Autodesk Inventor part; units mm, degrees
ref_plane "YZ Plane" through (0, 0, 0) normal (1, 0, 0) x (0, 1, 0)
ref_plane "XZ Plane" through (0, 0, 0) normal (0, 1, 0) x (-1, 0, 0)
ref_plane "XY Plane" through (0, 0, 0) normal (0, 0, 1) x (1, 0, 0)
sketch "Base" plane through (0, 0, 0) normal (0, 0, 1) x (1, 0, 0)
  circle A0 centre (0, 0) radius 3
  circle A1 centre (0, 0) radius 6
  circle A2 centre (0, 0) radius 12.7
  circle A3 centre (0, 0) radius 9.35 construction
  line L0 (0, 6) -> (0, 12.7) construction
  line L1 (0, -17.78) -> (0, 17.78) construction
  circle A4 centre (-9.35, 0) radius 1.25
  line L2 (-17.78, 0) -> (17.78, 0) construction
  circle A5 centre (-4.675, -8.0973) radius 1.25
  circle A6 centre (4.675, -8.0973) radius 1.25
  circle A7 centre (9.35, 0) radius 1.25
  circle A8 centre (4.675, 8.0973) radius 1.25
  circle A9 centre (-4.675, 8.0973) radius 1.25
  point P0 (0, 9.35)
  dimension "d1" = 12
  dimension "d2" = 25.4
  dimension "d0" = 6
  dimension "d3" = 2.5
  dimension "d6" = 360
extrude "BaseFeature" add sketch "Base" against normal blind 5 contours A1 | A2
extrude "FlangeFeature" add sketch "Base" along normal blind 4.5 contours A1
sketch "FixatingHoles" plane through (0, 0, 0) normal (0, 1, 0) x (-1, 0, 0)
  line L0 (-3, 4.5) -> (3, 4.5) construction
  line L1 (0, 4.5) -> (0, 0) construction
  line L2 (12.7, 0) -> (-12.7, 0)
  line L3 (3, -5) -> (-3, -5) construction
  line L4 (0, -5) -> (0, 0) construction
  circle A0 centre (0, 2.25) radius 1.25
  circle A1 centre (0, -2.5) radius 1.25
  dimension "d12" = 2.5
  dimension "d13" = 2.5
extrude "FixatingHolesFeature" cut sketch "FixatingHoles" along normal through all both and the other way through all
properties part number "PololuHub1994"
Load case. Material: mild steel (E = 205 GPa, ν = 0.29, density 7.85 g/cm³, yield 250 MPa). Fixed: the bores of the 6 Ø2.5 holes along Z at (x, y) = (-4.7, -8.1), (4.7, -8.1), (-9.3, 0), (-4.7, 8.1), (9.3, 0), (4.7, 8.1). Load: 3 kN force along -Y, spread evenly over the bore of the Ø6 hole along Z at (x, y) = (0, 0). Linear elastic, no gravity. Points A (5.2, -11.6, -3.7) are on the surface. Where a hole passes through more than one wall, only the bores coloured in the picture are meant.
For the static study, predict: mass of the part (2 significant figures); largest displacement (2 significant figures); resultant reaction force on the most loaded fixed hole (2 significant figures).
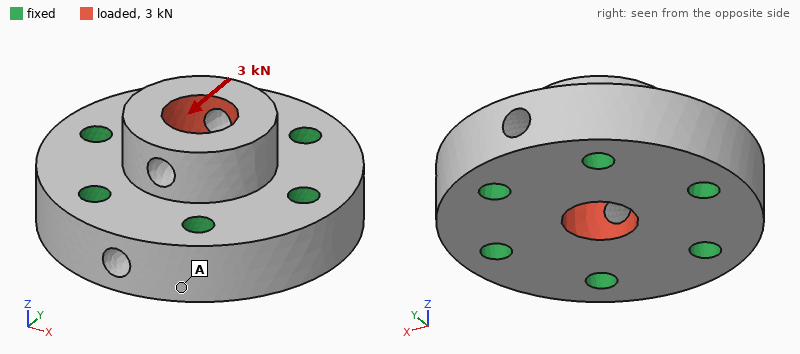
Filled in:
20 g
2.5 µm
690 N
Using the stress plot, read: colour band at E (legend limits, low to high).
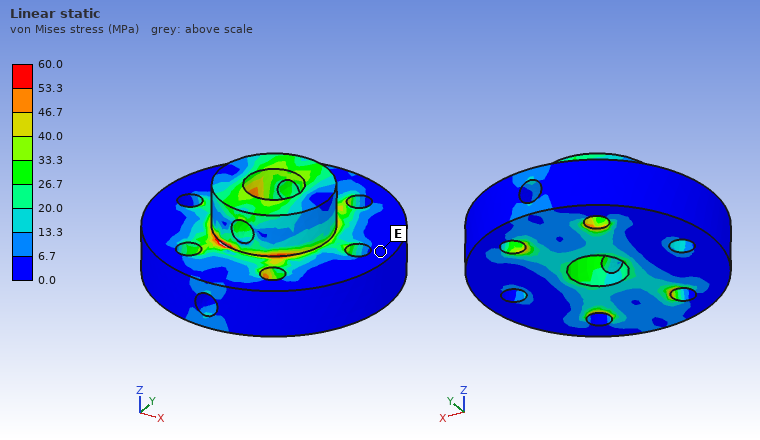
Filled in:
0.0 to 6.7 MPa
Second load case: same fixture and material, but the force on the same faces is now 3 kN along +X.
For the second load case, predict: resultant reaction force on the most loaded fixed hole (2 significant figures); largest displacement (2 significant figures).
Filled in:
860 N
2.9 µm
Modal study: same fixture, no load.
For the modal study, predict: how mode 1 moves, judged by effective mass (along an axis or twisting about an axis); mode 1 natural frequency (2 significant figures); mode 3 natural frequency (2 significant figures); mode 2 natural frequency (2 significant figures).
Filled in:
along X
86 kHz
90 kHz
89 kHz
